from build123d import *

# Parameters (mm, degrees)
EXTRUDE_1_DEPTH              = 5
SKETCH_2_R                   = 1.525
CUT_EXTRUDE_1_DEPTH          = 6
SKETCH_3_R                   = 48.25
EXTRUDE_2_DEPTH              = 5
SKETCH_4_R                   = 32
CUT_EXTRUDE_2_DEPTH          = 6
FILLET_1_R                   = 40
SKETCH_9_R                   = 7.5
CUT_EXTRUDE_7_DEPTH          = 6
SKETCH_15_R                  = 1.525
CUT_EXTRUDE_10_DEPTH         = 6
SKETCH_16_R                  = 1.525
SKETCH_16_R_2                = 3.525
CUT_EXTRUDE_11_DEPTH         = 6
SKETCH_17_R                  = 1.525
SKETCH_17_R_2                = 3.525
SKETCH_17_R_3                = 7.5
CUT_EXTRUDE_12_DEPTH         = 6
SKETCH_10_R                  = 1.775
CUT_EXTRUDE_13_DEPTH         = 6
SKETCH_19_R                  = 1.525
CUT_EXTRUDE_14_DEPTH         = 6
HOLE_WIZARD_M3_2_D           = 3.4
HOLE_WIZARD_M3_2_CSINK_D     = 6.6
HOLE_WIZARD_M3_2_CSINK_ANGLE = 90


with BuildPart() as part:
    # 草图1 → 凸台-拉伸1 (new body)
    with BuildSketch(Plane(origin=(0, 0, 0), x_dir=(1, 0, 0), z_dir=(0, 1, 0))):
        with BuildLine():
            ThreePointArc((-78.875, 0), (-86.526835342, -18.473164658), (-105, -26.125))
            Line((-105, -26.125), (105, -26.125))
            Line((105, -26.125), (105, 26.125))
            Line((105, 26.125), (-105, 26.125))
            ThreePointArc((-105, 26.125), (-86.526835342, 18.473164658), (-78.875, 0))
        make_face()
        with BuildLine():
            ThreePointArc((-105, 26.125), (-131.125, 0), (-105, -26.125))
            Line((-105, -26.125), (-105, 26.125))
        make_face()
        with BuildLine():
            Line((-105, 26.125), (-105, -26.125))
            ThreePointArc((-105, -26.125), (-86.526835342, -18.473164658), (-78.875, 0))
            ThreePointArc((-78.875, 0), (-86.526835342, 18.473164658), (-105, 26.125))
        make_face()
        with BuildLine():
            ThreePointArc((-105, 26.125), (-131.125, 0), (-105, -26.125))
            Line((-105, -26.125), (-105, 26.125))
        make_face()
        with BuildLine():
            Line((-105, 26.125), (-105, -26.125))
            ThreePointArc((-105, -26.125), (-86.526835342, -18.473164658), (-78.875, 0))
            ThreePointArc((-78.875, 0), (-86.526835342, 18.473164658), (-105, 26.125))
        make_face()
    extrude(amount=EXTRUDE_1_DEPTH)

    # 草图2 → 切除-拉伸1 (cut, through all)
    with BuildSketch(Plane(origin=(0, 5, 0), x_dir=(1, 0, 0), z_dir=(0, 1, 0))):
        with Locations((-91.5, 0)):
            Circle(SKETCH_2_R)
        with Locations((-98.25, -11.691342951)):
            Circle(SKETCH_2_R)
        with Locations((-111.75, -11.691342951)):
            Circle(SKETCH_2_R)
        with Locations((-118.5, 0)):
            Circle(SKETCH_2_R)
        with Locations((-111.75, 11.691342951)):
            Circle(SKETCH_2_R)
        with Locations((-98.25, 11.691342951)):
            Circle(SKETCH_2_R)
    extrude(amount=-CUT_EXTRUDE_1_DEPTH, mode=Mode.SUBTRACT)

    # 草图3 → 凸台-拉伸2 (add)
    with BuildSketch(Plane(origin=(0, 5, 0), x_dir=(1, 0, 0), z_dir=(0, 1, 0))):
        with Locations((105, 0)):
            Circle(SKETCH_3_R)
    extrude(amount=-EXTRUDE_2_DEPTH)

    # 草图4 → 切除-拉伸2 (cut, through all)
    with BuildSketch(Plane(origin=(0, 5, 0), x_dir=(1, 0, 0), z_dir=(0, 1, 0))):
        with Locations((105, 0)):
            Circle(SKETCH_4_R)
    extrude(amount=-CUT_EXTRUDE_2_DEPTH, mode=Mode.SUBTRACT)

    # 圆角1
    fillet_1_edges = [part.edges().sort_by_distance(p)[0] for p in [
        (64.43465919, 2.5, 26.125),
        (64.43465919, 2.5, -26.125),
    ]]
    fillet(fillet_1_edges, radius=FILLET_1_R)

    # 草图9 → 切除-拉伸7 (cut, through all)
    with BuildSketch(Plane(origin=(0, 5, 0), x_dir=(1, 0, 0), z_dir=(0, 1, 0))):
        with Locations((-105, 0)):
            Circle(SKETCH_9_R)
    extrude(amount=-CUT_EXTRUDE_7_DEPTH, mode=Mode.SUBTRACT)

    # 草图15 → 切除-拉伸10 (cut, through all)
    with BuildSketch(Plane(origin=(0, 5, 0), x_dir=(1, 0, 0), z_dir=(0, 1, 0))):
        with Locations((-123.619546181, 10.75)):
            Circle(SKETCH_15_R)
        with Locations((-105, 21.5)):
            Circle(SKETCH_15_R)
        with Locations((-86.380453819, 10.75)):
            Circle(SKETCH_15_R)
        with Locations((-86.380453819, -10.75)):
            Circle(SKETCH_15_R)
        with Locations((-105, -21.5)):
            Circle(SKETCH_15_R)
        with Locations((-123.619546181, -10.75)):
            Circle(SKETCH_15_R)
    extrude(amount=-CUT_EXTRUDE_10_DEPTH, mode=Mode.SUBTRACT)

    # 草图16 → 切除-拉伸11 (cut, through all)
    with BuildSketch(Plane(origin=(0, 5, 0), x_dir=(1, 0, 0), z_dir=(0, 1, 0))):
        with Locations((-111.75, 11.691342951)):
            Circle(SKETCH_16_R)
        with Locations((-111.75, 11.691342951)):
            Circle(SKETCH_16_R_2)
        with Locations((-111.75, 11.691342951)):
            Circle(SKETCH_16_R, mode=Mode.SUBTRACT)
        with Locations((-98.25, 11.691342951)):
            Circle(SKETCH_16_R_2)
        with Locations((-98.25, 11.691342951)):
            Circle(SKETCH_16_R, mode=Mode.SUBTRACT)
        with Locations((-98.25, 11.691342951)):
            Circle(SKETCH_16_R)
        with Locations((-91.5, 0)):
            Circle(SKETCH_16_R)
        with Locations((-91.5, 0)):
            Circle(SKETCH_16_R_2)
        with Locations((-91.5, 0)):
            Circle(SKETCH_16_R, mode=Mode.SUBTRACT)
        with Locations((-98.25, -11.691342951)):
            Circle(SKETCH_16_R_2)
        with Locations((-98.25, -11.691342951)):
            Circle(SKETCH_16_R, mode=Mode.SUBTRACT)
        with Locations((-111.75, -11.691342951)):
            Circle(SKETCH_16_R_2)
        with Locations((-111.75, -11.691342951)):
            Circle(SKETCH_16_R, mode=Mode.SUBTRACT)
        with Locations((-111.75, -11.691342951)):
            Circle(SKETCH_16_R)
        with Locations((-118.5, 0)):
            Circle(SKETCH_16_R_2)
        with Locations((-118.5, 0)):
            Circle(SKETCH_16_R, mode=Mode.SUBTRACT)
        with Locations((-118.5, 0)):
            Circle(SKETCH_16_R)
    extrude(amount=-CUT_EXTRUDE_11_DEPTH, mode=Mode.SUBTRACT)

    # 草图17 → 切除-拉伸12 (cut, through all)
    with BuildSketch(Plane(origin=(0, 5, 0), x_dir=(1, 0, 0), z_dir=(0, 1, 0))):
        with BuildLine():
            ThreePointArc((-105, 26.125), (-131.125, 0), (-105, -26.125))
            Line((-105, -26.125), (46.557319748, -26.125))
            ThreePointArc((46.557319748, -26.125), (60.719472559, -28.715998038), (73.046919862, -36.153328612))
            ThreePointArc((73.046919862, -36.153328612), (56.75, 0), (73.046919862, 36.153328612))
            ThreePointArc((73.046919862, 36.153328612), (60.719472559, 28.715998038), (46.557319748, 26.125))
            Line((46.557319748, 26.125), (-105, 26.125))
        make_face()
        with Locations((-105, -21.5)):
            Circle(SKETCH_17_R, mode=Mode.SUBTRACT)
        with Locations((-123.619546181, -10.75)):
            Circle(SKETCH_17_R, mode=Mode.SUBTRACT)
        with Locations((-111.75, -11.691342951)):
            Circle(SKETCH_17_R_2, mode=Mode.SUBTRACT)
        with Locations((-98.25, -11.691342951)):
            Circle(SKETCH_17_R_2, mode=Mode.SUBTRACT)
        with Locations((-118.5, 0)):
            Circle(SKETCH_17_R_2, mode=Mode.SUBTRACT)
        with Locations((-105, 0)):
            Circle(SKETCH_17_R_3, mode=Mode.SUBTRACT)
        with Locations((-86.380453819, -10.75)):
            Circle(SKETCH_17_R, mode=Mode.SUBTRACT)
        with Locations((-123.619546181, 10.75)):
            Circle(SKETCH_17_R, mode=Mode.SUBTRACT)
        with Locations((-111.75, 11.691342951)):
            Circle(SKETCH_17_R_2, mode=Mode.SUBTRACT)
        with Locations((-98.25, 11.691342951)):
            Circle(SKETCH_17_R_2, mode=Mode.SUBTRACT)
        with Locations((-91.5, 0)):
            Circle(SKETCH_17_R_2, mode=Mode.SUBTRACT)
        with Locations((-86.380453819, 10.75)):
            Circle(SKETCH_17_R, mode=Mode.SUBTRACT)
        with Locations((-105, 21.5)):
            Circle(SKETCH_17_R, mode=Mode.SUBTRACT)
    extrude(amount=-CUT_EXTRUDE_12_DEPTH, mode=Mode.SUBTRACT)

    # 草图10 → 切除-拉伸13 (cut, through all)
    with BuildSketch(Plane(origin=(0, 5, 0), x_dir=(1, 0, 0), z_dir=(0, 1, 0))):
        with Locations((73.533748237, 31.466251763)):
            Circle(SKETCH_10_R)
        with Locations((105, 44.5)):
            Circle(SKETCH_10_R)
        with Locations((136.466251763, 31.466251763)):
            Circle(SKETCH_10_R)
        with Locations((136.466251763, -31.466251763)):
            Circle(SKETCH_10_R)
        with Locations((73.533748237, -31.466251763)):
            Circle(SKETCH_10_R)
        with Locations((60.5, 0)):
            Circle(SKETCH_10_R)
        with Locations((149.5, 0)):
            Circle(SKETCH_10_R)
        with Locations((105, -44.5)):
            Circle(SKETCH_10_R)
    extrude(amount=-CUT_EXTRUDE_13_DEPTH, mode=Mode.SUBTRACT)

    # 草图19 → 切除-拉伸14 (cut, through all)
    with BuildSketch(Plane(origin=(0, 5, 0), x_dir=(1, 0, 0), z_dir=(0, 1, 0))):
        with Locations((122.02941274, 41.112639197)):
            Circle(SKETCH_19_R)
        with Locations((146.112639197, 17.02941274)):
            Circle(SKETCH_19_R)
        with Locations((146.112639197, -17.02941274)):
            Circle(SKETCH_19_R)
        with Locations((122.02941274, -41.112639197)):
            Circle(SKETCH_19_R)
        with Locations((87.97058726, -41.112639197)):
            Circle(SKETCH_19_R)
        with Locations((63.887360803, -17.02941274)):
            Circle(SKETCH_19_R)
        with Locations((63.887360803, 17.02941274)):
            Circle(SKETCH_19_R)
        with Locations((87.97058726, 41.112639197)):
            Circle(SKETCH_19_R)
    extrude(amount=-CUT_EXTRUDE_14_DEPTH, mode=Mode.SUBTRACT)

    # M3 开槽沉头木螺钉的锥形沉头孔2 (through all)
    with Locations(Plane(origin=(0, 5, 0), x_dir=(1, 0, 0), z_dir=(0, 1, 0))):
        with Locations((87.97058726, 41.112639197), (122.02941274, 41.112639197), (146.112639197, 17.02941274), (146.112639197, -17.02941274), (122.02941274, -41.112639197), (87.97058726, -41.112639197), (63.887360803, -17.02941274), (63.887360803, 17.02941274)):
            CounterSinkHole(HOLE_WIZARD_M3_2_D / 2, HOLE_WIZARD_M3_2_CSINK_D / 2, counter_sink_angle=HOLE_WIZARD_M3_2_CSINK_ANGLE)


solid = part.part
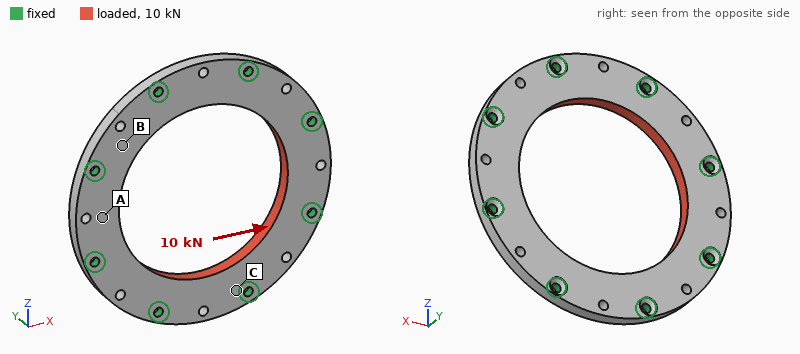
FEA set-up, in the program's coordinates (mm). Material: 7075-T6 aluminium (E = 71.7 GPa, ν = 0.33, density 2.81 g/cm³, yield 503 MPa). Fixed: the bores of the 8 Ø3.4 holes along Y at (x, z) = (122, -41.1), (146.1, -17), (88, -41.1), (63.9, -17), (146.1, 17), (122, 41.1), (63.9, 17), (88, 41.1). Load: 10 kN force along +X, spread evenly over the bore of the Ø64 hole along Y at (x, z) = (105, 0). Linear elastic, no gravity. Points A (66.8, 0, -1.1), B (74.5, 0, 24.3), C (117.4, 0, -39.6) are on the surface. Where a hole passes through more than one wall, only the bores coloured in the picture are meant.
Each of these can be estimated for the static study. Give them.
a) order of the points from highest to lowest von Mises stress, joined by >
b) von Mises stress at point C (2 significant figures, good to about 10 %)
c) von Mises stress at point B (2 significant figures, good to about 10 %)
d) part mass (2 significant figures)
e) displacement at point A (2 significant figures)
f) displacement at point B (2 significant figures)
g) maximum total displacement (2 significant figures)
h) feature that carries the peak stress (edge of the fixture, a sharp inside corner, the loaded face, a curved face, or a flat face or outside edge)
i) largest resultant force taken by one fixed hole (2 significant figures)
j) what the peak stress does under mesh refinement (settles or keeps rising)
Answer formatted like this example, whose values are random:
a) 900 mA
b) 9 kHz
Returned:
a) C > B > A
b) 24 MPa
c) 14 MPa
d) 55 g
e) 5.8 µm
f) 4.1 µm
g) 8.6 µm
h) edge of the fixture
i) 1.5 kN
j) keeps rising
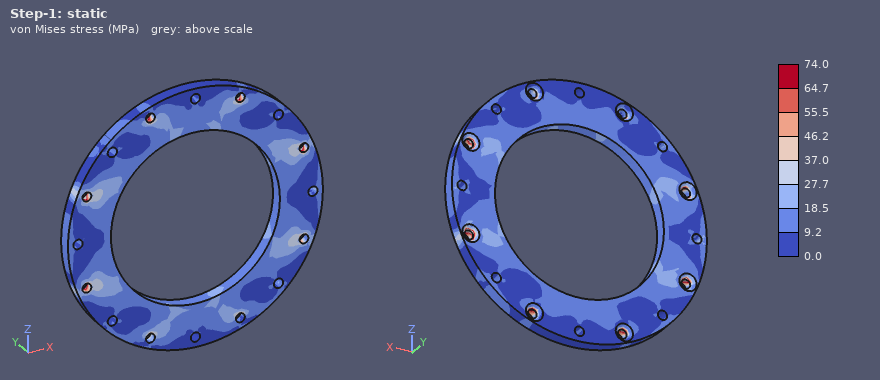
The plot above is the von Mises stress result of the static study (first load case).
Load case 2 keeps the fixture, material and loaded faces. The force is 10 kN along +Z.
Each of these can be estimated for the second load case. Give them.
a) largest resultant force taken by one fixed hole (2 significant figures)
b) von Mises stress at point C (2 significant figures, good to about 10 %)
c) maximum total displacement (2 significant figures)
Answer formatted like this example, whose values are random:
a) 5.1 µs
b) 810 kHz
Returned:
a) 1.5 kN
b) 18 MPa
c) 8.6 µm
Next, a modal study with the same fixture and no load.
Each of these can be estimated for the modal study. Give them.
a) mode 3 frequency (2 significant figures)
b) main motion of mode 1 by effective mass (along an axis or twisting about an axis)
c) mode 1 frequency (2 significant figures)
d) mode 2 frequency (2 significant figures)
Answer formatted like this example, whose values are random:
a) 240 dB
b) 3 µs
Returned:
a) 15 kHz
b) along Y
c) 13 kHz
d) 15 kHz
